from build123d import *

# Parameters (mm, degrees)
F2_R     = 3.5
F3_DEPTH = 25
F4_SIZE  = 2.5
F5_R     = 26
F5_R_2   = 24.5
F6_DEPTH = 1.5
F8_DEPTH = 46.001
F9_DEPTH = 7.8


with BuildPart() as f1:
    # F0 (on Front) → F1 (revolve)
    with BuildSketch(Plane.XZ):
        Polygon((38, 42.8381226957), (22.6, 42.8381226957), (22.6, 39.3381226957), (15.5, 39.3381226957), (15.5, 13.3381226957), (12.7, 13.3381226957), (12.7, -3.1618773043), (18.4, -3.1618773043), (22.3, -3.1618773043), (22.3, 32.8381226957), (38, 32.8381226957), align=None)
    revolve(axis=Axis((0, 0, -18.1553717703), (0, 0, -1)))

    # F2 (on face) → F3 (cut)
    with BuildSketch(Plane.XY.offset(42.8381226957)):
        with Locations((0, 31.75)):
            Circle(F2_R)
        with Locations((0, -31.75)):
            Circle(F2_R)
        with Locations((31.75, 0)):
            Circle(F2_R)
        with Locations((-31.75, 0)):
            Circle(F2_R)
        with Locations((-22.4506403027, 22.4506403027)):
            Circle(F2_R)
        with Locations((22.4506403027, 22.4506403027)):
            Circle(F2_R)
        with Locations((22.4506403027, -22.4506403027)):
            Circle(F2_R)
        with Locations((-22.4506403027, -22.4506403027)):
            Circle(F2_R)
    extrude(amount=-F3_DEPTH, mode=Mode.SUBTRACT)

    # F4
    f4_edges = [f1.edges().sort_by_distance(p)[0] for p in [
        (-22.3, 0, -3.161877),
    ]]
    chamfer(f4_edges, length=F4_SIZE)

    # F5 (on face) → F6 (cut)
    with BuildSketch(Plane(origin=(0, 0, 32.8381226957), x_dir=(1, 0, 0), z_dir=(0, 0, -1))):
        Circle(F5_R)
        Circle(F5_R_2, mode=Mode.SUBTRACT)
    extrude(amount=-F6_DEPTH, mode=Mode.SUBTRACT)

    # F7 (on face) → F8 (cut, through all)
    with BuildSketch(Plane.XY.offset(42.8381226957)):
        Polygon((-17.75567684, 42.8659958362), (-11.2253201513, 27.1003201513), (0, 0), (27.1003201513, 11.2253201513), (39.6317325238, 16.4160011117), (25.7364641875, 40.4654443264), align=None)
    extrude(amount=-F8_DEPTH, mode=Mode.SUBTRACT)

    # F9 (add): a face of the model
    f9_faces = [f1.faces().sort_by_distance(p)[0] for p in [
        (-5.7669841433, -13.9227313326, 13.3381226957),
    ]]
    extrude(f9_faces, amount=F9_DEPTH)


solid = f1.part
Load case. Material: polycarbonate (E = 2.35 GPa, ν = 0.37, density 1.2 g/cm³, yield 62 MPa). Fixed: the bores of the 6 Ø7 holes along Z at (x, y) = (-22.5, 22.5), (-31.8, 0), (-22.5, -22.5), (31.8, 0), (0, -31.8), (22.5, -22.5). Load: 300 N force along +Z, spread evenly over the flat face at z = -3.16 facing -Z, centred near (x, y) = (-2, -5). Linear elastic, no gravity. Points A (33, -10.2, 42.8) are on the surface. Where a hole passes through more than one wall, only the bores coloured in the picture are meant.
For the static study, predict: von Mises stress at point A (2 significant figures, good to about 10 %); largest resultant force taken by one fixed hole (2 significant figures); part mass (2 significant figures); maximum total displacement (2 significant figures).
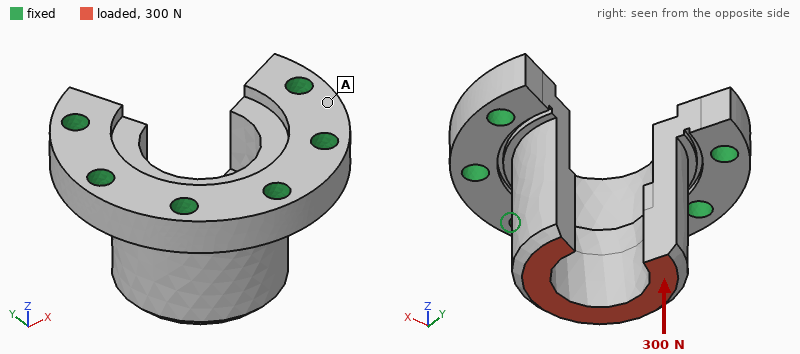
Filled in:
0.22 MPa
66 N
59 g
29 µm
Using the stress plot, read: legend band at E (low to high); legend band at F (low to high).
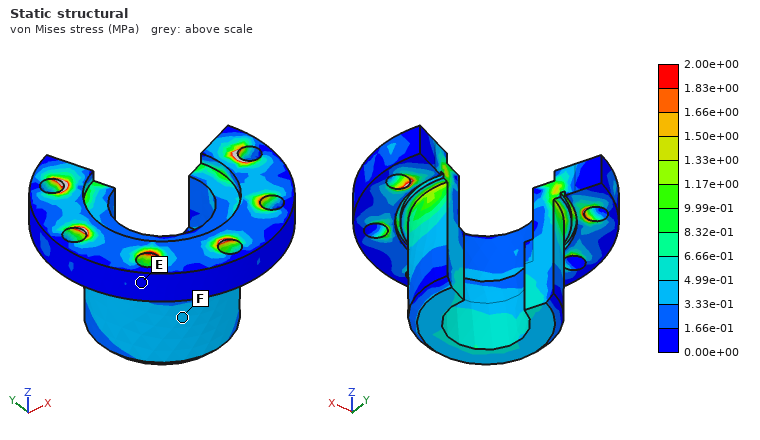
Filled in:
0.00e+00 to 1.66e-01 MPa
3.33e-01 to 4.99e-01 MPa
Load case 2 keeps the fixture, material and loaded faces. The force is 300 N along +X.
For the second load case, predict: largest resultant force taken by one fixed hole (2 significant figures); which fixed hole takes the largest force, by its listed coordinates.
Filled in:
210 N
(-31.8, 0)
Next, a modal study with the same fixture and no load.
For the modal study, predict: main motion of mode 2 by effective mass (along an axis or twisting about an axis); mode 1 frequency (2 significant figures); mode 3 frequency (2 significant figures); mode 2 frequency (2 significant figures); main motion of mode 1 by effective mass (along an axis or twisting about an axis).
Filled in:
along Y
1600 Hz
2500 Hz
2100 Hz
along X
